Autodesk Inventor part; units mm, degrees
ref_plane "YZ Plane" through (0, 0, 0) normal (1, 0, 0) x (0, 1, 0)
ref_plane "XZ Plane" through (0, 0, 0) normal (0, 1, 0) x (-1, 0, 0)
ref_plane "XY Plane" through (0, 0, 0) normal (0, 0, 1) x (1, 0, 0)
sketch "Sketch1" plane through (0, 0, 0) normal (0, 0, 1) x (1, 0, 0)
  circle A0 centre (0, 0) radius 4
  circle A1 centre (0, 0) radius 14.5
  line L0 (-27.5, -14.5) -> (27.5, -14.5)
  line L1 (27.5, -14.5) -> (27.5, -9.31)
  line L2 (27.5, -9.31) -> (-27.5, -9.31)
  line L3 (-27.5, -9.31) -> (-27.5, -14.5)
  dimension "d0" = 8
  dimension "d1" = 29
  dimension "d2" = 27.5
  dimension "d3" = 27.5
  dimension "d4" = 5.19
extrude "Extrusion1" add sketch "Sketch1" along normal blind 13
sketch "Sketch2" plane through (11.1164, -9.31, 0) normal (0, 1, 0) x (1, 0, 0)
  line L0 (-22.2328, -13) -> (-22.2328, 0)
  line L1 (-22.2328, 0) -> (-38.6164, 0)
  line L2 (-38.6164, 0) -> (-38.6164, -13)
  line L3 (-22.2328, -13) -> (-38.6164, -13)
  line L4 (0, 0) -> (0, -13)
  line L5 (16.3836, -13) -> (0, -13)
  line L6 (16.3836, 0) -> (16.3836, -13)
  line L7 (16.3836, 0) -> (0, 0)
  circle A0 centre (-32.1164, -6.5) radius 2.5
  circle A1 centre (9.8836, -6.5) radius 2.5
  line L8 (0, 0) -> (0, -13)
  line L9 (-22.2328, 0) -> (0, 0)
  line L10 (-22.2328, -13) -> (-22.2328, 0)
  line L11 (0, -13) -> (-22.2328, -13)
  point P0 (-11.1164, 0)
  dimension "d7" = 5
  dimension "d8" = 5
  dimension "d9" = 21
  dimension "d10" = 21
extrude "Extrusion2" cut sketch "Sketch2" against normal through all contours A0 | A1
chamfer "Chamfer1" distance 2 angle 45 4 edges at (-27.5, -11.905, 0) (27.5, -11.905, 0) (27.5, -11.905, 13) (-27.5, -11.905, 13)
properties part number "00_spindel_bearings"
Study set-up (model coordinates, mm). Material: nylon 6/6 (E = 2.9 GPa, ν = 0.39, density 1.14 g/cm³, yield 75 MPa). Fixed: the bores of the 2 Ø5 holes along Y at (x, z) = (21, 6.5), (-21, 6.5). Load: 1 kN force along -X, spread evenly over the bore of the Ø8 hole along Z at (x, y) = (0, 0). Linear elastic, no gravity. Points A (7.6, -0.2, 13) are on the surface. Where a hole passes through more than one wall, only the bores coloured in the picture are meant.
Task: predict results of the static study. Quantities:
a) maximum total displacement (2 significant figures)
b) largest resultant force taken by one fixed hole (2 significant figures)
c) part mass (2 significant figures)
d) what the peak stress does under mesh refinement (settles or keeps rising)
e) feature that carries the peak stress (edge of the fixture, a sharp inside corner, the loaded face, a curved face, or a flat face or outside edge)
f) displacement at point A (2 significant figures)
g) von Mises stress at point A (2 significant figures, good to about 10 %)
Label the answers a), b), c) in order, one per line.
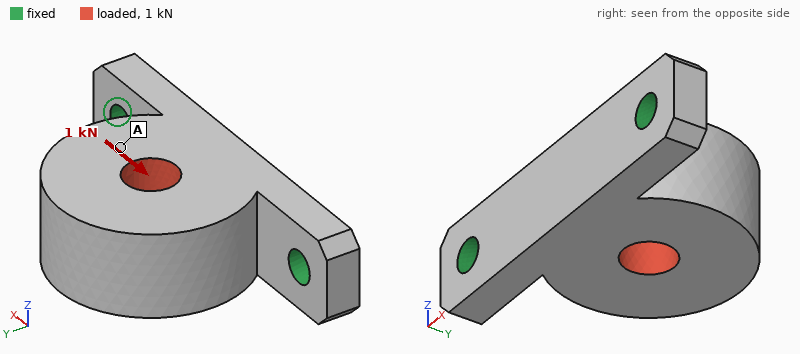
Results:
a) 0.35 mm
b) 630 N
c) 12 g
d) keeps rising
e) edge of the fixture
f) 0.20 mm
g) 6.3 MPa
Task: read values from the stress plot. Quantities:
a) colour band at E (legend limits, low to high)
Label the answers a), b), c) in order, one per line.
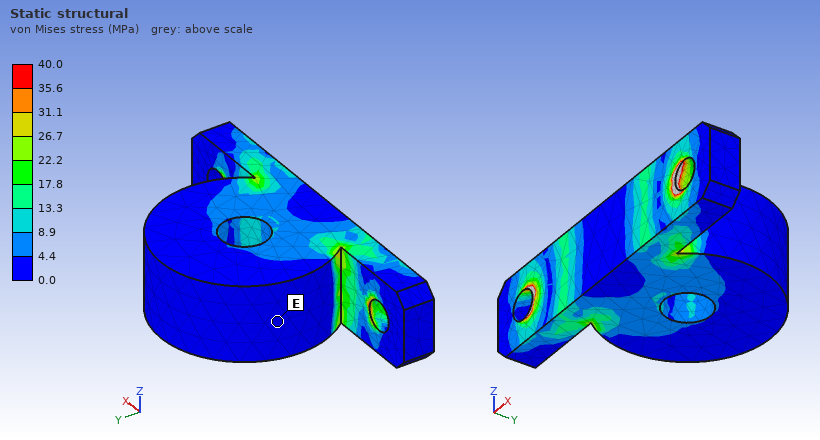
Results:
a) 0.0 to 4.4 MPa
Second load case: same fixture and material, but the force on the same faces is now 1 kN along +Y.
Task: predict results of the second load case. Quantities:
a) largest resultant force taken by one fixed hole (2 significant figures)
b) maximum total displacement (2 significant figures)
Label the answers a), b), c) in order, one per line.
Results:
a) 540 N
b) 0.24 mm
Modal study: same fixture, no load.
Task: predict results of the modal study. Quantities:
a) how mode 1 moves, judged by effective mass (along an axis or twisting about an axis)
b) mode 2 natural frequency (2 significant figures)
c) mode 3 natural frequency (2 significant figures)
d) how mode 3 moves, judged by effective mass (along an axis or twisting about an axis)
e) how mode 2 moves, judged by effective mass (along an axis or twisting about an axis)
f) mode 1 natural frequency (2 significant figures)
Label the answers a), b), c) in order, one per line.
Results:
a) along Z
b) 3100 Hz
c) 3400 Hz
d) along Y
e) along X
f) 1200 Hz
